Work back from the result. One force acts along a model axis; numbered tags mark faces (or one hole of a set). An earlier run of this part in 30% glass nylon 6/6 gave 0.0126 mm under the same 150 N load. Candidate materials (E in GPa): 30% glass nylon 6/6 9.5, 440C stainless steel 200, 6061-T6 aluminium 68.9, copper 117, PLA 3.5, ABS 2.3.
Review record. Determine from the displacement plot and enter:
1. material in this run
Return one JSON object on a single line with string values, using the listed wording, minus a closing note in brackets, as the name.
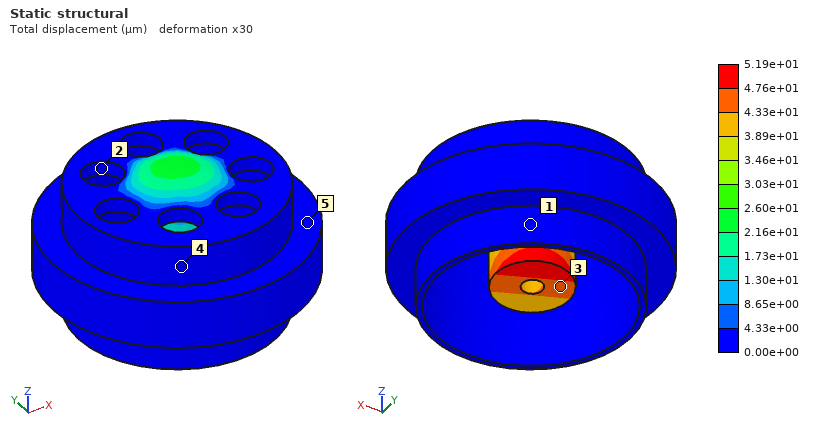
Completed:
{"material in this run": "ABS"}
